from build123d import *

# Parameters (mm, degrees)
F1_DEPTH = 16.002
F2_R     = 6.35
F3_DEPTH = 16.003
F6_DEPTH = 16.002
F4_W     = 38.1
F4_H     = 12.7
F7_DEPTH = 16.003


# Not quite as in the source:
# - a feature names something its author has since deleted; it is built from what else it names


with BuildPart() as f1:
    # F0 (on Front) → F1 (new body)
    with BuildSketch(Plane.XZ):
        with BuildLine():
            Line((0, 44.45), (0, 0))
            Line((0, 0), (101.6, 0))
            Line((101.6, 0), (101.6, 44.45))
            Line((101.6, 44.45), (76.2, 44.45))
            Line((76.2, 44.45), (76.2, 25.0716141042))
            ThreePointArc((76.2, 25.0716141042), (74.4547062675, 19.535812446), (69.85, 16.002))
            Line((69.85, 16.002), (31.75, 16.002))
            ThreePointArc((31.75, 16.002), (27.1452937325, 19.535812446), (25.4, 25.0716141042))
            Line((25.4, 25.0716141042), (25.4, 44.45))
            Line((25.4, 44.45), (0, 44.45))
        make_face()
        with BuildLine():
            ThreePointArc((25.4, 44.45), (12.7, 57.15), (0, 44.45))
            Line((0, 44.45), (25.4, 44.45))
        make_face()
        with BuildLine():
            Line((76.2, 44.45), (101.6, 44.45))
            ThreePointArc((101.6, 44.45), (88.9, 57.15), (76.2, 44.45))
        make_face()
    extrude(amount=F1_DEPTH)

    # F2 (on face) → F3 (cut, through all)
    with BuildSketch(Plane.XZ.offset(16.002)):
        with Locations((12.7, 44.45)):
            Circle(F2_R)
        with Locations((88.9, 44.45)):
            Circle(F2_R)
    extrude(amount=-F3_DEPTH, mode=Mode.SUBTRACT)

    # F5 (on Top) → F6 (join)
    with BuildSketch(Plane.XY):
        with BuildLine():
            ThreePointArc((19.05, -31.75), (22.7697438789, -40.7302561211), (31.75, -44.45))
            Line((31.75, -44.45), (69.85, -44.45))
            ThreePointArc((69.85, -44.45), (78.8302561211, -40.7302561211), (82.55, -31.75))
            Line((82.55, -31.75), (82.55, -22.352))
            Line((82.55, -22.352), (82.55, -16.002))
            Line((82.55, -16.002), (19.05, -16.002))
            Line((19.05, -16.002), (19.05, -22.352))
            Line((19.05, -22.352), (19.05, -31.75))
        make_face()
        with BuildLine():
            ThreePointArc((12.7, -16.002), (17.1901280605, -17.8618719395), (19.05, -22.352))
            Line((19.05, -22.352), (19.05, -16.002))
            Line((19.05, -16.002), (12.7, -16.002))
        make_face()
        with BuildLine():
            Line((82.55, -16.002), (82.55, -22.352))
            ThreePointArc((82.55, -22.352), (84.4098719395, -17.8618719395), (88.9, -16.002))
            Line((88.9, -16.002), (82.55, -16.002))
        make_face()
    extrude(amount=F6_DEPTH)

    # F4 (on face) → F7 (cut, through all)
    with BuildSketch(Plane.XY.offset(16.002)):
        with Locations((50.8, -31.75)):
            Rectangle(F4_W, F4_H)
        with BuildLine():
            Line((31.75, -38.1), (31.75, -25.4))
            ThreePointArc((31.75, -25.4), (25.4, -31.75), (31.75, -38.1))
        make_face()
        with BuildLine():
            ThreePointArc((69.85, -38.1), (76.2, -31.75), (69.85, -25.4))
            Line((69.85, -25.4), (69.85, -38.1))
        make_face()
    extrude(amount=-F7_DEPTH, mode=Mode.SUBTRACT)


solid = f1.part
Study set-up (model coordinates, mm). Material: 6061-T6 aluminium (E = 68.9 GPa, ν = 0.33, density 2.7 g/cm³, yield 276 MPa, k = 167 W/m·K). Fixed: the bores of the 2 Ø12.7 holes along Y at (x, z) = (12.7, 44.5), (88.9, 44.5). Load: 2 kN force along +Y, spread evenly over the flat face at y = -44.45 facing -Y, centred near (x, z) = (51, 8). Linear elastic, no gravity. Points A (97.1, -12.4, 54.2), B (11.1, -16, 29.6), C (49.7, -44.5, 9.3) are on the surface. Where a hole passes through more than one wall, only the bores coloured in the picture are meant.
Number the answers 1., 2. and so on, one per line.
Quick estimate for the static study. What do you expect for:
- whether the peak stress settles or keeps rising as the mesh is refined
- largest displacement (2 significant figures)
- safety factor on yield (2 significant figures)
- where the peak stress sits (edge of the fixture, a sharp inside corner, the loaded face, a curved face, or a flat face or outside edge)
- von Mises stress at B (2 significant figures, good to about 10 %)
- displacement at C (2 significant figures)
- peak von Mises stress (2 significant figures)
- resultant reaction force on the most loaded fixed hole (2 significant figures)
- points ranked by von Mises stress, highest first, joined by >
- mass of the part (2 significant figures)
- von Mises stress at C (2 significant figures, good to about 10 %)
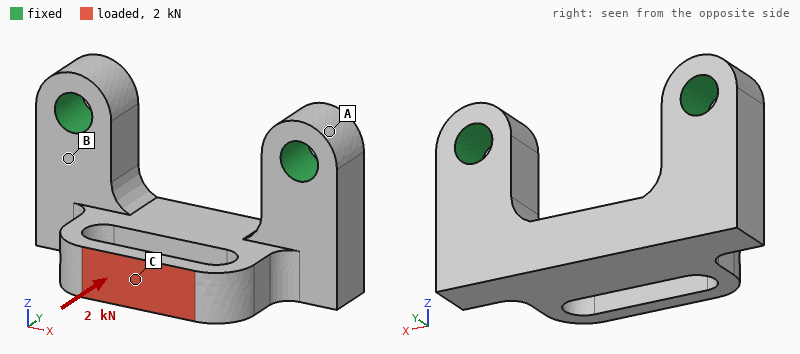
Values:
1. settles
2. 0.11 mm
3. 3.0
4. a curved face
5. 21 MPa
6. 0.096 mm
7. 92 MPa
8. 1.0 kN
9. C > B > A
10. 190 g
11. 69 MPa
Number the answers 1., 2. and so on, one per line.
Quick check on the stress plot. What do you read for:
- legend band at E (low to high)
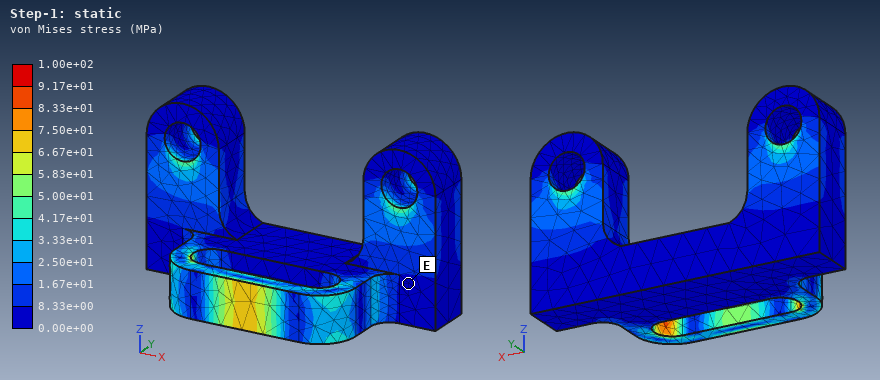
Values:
1. 0.00e+00 to 8.33e+00 MPa
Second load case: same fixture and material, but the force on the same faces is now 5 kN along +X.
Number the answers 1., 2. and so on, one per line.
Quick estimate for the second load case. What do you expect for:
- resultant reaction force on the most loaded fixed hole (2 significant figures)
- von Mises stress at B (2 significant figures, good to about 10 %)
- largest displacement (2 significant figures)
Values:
1. 3.5 kN
2. 35 MPa
3. 0.14 mm
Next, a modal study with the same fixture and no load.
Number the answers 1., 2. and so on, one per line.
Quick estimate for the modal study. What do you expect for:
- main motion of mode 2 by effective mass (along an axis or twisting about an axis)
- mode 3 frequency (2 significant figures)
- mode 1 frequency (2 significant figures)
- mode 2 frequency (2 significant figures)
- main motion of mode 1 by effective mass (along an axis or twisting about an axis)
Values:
1. along X
2. 6900 Hz
3. 3300 Hz
4. 5700 Hz
5. along Y
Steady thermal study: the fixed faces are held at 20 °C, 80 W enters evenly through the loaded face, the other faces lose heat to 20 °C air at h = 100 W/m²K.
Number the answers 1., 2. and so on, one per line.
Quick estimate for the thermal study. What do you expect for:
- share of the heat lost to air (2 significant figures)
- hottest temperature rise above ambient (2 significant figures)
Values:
1. 36 %
2. 85 K
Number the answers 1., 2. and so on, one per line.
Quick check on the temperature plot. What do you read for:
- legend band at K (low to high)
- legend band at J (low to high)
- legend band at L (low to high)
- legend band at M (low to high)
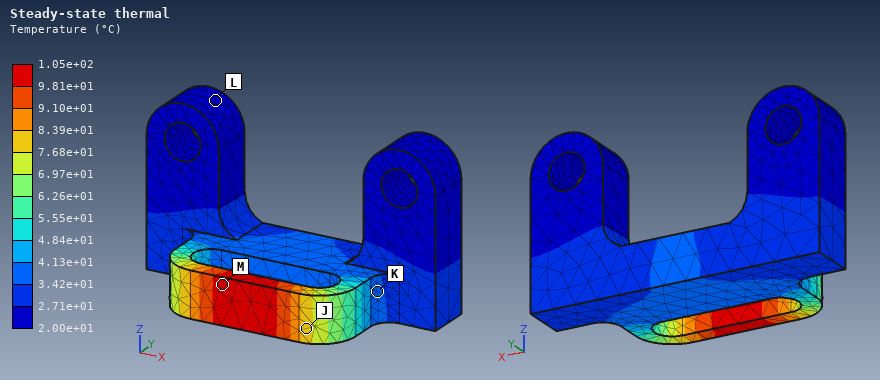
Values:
1. 3.42e+01 to 4.13e+01 °C
2. 7.68e+01 to 8.39e+01 °C
3. 2.00e+01 to 2.71e+01 °C
4. 9.81e+01 to 1.05e+02 °C
